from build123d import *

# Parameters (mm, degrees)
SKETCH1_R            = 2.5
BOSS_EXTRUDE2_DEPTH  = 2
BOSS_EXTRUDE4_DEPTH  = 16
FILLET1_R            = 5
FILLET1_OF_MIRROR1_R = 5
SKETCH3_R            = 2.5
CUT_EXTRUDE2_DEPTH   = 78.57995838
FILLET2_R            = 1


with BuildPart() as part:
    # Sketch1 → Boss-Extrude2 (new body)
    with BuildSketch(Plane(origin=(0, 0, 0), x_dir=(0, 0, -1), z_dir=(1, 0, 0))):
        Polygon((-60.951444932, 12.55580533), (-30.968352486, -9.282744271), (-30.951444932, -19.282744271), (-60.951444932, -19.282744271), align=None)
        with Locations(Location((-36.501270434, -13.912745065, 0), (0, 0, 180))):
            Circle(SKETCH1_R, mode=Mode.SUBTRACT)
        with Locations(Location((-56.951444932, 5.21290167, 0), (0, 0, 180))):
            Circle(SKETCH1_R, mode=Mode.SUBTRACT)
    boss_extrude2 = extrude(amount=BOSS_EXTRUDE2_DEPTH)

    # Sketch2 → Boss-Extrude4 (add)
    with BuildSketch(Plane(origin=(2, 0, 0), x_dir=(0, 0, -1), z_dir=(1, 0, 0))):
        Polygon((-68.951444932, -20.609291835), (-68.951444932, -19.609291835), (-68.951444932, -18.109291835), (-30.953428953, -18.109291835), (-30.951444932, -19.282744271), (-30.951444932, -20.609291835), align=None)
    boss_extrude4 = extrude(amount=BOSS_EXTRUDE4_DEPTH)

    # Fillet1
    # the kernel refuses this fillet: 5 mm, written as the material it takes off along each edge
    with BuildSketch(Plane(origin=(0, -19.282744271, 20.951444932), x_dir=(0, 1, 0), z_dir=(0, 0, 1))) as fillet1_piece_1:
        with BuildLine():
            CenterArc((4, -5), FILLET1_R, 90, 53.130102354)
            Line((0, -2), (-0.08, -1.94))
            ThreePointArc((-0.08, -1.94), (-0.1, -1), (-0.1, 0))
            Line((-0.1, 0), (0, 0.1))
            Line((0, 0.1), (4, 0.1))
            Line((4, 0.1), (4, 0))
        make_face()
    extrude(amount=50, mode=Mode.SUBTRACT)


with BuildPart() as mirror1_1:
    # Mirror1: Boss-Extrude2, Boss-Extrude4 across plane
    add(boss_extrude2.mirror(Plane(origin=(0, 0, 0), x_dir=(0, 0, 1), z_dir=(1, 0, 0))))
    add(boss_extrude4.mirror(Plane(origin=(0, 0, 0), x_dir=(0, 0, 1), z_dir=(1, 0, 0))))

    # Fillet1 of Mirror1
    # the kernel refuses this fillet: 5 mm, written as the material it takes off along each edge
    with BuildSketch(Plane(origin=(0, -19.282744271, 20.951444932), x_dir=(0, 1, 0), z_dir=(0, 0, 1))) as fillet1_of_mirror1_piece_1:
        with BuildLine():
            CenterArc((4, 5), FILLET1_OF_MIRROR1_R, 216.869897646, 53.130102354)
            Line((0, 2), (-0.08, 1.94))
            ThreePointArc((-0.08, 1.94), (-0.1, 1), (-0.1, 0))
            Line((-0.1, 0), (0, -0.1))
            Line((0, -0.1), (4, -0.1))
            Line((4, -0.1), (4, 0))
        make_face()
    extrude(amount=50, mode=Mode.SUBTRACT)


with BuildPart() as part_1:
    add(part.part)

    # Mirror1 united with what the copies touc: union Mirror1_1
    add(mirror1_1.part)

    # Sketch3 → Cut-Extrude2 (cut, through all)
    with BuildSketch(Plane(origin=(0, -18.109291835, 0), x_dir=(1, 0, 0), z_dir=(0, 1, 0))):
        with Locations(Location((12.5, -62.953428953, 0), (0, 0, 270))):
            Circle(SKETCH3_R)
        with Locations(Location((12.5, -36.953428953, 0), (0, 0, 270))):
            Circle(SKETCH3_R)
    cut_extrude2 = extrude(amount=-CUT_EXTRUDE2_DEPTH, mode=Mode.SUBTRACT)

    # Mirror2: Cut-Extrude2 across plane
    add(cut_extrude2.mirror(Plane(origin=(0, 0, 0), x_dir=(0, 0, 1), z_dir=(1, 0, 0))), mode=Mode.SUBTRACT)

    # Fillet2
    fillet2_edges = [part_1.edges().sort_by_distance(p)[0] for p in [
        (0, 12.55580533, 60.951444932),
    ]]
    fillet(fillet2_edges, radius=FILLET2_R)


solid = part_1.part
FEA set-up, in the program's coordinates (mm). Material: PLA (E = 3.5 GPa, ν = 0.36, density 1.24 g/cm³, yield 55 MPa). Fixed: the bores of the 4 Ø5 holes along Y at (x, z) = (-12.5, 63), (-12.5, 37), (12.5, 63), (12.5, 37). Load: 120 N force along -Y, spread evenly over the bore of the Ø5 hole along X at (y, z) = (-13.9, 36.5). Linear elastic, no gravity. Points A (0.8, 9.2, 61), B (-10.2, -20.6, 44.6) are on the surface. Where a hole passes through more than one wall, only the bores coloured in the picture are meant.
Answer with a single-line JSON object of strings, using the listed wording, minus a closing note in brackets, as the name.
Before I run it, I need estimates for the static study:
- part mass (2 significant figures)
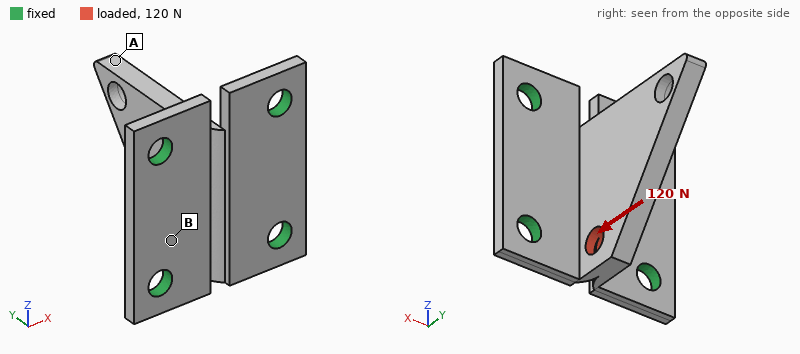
{"part mass": "6.3 g"}
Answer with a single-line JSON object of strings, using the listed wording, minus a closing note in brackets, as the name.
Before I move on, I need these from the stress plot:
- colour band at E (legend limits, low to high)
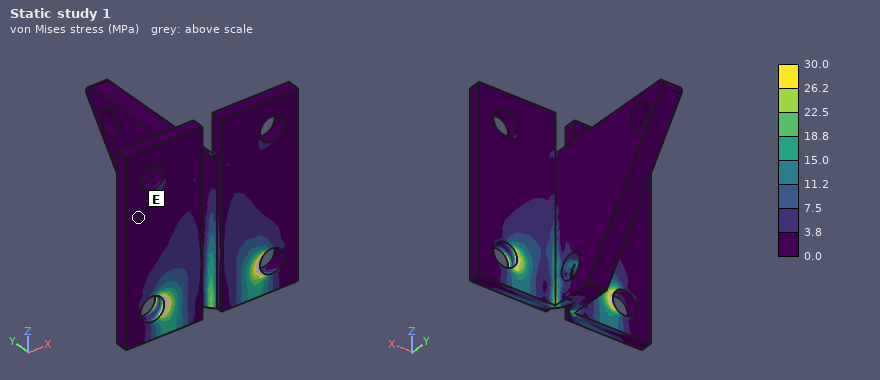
{"colour band at E": "0.0 to 3.8 MPa"}
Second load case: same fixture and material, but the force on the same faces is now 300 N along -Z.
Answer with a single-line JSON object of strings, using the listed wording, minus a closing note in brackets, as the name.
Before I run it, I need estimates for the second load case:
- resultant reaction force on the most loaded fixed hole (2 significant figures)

{"resultant reaction force on the most loaded fixed hole": "110 N"}
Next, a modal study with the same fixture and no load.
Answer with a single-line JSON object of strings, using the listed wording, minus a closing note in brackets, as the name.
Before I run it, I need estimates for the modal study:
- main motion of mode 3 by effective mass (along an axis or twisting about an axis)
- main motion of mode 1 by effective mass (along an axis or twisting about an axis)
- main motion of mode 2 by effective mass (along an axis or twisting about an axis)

{"main motion of mode 3 by effective mass": "along Y", "main motion of mode 1 by effective mass": "along X", "main motion of mode 2 by effective mass": "along Z"}
